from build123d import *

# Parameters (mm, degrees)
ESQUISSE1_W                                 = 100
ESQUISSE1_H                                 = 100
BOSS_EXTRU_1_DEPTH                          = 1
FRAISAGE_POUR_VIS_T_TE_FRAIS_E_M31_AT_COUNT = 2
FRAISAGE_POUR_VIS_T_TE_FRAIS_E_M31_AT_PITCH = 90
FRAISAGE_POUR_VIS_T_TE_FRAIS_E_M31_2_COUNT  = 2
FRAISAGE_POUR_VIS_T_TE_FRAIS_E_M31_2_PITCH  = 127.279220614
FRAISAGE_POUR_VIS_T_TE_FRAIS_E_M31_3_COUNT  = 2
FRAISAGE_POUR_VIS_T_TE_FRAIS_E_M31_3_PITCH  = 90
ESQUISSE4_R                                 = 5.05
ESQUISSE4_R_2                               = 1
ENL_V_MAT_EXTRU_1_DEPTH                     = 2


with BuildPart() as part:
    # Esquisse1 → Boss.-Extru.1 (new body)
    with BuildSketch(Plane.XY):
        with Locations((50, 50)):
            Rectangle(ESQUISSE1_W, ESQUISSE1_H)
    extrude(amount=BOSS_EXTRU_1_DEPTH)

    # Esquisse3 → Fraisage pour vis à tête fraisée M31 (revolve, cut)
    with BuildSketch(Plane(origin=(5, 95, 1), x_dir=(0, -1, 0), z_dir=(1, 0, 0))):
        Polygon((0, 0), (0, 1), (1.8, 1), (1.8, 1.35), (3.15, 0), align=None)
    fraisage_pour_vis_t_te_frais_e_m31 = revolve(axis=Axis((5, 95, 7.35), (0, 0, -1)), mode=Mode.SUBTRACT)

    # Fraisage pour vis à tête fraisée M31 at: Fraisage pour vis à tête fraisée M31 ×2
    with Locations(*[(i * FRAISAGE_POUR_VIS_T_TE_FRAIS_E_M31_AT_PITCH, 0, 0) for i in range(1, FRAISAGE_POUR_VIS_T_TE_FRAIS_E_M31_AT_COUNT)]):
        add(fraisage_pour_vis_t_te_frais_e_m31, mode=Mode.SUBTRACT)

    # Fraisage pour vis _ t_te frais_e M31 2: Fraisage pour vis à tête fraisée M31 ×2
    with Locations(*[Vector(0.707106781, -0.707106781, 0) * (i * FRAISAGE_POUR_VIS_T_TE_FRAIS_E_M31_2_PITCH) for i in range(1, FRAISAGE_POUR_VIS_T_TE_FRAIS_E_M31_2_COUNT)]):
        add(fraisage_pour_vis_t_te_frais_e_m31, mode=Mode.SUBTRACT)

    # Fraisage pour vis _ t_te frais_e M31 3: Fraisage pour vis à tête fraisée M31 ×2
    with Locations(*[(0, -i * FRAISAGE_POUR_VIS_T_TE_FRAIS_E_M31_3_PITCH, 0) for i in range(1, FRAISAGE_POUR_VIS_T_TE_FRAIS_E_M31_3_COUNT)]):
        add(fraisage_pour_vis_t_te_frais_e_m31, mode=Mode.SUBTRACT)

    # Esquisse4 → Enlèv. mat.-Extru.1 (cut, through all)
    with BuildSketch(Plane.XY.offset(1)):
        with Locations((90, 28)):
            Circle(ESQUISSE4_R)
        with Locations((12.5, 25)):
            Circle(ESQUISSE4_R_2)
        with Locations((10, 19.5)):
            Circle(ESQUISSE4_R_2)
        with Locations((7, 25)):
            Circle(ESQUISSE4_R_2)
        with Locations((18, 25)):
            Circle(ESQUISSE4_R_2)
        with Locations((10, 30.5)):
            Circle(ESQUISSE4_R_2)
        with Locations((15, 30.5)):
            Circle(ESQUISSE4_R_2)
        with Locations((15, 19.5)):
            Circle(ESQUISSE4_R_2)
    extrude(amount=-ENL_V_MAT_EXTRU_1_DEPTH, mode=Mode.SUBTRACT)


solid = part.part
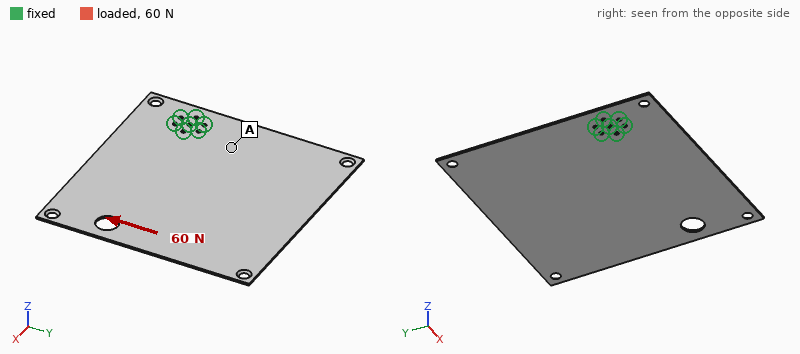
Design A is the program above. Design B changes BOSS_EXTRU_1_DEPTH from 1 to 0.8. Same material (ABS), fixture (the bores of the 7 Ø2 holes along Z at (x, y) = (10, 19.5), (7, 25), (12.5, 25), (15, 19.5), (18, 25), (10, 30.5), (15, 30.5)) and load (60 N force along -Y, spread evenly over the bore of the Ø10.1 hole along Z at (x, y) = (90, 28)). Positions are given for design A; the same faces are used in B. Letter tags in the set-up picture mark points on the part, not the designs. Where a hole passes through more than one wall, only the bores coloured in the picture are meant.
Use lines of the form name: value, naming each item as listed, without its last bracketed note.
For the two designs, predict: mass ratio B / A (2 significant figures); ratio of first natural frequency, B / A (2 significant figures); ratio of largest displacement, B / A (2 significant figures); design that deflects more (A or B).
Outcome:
mass ratio B / A: 0.80
ratio of first natural frequency, B / A: 0.80
ratio of largest displacement, B / A: 1.2
design that deflects more: B
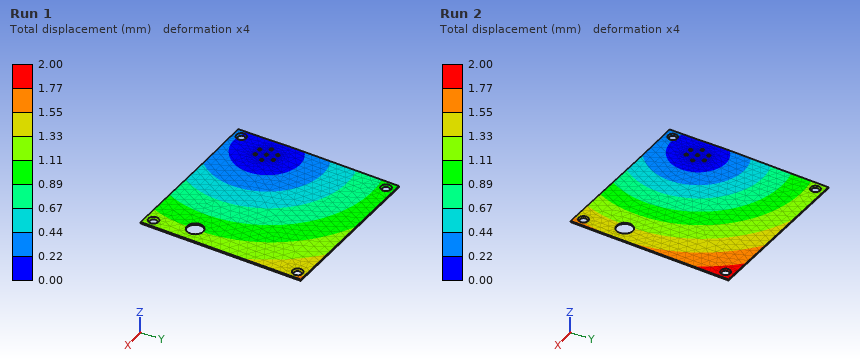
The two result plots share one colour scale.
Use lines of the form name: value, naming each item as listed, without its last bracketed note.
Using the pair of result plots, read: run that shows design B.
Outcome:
run that shows design B: Run 2
